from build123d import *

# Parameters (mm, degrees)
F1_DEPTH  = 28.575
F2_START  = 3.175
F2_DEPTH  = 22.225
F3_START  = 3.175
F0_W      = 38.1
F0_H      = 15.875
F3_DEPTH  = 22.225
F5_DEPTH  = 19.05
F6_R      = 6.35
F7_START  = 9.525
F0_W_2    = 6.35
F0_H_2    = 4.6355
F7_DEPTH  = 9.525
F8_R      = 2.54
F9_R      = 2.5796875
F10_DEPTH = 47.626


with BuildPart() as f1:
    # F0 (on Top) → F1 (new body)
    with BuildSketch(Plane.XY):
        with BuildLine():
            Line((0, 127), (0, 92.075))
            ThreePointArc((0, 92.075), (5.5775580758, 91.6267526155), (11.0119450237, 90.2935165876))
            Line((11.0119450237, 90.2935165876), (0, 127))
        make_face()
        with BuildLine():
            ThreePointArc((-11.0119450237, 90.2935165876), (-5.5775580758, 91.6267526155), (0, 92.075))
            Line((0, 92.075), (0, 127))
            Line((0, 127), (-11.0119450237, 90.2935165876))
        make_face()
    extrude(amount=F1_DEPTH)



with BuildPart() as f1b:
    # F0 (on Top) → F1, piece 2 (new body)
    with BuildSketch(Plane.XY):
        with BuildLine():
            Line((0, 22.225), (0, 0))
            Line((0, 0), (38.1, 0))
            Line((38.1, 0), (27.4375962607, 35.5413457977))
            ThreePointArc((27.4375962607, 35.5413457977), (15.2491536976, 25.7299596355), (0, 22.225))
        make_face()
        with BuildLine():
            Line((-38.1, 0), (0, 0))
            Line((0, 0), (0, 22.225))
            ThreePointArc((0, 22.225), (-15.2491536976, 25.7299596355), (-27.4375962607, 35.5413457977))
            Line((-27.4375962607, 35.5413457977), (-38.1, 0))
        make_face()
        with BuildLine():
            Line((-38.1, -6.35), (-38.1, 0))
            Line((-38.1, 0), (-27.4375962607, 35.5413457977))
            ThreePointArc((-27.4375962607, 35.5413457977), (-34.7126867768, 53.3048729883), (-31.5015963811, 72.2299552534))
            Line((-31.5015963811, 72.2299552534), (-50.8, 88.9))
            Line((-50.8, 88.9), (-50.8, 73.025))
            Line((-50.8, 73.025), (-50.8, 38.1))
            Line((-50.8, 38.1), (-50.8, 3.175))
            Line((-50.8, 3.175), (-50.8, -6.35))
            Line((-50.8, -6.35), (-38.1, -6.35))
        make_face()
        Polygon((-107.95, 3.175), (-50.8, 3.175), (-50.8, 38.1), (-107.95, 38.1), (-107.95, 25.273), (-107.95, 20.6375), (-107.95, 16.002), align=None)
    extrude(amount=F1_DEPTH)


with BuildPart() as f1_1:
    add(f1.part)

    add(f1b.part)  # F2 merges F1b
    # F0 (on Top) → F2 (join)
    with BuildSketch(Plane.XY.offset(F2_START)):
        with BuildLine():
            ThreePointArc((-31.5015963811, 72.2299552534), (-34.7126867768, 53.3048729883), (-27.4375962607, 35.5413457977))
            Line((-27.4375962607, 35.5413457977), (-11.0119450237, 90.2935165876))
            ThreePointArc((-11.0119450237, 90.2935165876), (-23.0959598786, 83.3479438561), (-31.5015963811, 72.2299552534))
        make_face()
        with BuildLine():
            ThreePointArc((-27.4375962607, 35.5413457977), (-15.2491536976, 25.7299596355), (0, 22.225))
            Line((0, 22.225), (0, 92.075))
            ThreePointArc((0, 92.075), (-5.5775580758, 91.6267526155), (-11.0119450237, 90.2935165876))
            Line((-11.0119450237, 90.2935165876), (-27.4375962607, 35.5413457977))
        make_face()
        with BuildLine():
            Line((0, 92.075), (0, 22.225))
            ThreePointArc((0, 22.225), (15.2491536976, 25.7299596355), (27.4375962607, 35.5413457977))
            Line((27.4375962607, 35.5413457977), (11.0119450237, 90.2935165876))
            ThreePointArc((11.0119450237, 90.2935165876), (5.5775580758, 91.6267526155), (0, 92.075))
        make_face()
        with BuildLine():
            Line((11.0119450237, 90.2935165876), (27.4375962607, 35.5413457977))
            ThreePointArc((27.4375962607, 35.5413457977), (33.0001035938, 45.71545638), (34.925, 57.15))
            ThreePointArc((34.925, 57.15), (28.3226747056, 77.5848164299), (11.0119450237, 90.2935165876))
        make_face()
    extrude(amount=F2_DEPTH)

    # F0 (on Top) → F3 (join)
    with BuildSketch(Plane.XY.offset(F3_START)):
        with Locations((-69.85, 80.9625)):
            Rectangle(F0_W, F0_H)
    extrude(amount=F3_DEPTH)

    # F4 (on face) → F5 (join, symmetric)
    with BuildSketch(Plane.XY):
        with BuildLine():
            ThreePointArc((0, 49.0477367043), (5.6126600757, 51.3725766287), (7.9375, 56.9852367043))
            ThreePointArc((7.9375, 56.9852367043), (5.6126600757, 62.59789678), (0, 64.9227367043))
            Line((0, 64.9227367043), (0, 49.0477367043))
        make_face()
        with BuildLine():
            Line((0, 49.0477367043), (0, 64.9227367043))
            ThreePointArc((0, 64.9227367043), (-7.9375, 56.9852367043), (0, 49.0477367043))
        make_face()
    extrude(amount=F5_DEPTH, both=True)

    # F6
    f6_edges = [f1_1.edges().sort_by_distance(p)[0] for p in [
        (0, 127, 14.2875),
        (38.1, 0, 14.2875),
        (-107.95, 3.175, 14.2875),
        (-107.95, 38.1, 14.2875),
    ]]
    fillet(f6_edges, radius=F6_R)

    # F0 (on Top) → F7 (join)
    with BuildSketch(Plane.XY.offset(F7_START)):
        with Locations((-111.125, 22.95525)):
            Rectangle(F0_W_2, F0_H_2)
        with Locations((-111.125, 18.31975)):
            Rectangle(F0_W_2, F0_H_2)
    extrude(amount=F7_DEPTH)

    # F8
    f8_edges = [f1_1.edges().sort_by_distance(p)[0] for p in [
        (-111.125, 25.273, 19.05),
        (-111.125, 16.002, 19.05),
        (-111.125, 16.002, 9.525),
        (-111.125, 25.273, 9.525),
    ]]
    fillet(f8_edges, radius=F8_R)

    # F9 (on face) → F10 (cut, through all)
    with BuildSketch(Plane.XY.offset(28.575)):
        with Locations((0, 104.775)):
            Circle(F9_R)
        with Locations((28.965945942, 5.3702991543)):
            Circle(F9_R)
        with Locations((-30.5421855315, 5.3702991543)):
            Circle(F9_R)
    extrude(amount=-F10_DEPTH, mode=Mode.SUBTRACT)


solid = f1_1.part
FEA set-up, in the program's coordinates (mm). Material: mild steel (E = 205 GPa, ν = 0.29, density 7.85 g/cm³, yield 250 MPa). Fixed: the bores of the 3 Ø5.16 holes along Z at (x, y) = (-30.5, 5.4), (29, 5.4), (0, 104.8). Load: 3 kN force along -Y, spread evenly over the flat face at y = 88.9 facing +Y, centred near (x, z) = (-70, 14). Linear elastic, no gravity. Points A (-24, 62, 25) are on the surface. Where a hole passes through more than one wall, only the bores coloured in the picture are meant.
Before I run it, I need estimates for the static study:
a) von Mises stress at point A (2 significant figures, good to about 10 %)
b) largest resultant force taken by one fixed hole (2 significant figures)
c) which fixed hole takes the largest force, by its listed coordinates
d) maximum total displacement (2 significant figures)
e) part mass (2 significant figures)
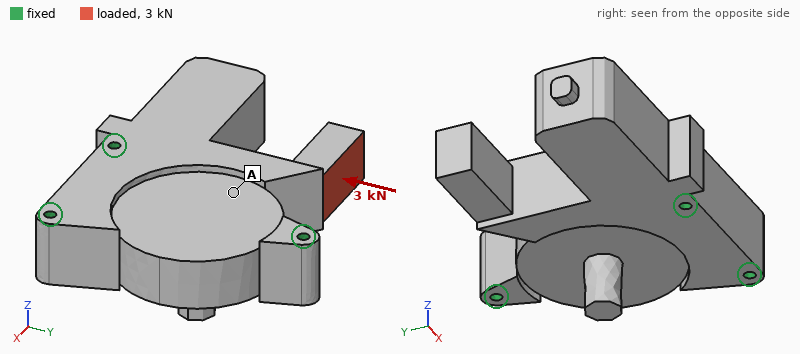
8.4 MPa
3.4 kN
(-30.5, 5.4)
71 µm
2.1 kg
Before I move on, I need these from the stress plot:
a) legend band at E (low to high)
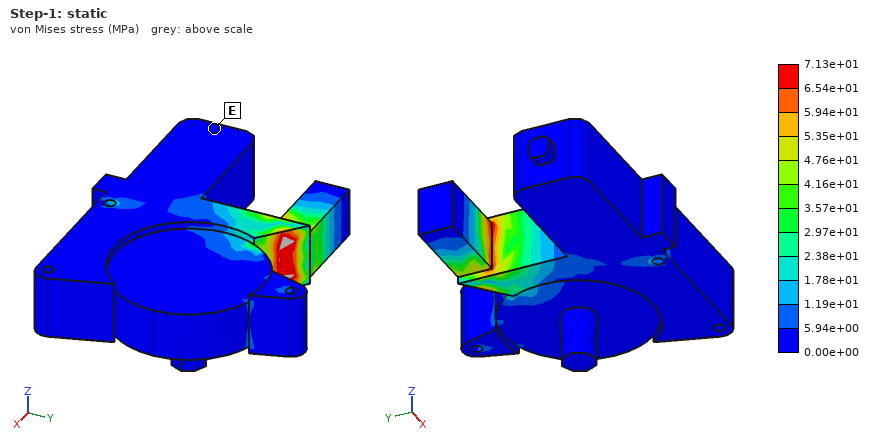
0.00e+00 to 5.94e+00 MPa
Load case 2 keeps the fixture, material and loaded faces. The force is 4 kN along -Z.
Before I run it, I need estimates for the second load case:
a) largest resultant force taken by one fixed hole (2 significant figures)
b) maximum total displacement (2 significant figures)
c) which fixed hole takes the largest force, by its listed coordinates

3.4 kN
0.11 mm
(-30.5, 5.4)
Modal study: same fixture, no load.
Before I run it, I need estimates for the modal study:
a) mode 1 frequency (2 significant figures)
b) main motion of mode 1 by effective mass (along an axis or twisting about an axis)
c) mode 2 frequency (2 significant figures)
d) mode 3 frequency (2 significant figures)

2800 Hz
along Z
3700 Hz
3700 Hz
